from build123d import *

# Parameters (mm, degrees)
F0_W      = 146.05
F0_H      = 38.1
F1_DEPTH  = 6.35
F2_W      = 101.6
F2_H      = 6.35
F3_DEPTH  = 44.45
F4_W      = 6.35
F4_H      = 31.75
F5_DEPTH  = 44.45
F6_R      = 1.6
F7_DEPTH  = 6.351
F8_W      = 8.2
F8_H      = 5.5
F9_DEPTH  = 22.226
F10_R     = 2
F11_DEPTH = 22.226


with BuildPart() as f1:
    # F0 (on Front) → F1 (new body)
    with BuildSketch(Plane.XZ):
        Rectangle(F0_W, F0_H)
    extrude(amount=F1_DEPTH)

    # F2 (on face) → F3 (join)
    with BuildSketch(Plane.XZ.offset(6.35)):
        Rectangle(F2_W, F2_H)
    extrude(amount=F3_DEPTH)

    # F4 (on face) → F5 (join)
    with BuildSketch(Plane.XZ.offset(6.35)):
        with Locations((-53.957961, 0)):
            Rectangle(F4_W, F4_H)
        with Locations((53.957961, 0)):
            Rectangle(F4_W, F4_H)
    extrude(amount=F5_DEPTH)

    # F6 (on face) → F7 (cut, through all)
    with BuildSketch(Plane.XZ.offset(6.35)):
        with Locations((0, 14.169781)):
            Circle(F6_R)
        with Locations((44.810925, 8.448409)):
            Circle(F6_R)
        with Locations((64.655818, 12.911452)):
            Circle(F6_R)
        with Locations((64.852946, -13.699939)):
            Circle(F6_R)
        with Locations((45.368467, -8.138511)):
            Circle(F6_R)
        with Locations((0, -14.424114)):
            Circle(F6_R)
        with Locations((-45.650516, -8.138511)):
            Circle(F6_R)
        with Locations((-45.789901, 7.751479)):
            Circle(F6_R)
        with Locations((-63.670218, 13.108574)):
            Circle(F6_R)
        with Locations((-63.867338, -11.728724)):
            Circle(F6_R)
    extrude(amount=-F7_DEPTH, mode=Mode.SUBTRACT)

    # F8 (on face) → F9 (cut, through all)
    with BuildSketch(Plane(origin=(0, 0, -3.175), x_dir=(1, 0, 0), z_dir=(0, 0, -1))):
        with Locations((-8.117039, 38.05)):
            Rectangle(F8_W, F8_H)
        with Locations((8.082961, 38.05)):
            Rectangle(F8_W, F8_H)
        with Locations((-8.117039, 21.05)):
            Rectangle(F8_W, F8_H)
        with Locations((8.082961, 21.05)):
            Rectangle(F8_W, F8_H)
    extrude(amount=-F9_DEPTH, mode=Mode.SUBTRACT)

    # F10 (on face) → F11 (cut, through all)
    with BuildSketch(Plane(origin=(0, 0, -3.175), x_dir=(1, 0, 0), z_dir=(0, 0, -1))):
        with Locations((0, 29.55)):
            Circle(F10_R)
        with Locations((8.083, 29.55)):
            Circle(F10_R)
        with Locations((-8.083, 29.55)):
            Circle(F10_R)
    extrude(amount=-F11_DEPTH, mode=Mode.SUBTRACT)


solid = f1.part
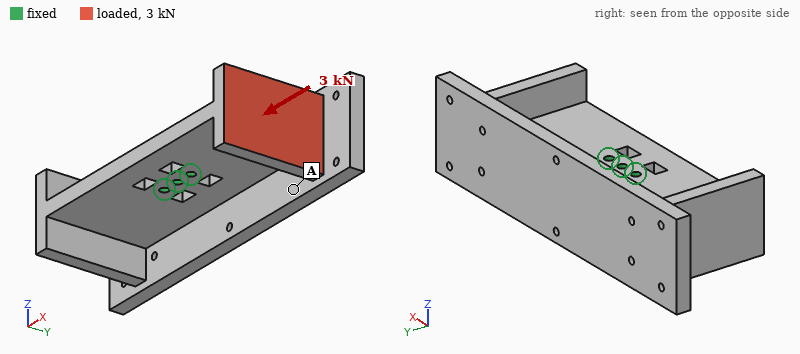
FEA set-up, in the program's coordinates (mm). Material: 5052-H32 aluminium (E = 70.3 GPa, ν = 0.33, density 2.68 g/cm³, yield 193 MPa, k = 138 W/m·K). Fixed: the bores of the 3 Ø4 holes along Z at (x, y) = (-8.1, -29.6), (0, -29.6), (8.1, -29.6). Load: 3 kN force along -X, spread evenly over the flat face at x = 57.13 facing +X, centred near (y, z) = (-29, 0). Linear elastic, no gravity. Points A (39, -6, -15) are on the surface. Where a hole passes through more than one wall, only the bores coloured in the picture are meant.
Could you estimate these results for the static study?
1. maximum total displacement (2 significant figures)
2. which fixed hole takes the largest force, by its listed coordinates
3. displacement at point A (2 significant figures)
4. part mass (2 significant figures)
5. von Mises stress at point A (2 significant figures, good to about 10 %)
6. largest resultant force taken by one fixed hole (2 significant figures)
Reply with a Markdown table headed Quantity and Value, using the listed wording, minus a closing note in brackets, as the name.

| Quantity | Value |
|---|---|
| maximum total displacement | 18 µm |
| which fixed hole takes the largest force, by its listed coordinates | (8.1, -29.6) |
| displacement at point A | 6.5 µm |
| part mass | 210 g |
| von Mises stress at point A | 3.7 MPa |
| largest resultant force taken by one fixed hole | 1.8 kN |
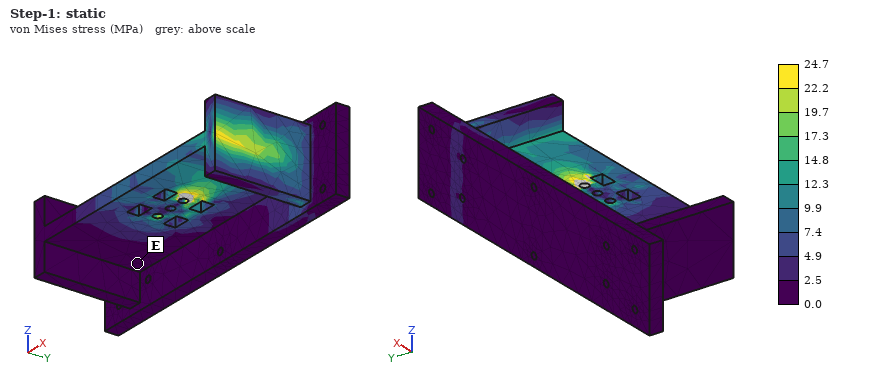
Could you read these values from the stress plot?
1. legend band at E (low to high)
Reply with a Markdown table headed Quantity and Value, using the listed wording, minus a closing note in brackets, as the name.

| Quantity | Value |
|---|---|
| legend band at E | 0.0 to 2.5 MPa |
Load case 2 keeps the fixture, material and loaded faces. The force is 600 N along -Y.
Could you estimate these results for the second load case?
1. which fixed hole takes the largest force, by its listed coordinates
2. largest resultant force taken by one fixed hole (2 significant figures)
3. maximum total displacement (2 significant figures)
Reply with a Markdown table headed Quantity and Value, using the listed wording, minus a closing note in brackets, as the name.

| Quantity | Value |
|---|---|
| which fixed hole takes the largest force, by its listed coordinates | (8.1, -29.6) |
| largest resultant force taken by one fixed hole | 1.8 kN |
| maximum total displacement | 54 µm |
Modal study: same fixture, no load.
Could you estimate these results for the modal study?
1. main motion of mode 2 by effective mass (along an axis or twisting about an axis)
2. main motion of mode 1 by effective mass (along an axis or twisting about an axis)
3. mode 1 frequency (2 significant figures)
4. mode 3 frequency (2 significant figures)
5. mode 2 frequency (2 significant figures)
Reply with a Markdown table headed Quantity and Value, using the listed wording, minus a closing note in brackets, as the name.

| Quantity | Value |
|---|---|
| main motion of mode 2 by effective mass | along Z |
| main motion of mode 1 by effective mass | twisting about Y |
| mode 1 frequency | 900 Hz |
| mode 3 frequency | 1800 Hz |
| mode 2 frequency | 1300 Hz |
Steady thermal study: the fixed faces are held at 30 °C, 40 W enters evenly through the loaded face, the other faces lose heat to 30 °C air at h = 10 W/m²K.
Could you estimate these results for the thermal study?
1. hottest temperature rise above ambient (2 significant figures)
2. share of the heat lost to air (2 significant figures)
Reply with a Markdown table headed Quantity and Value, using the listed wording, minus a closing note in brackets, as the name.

| Quantity | Value |
|---|---|
| hottest temperature rise above ambient | 43 K |
| share of the heat lost to air | 12 % |
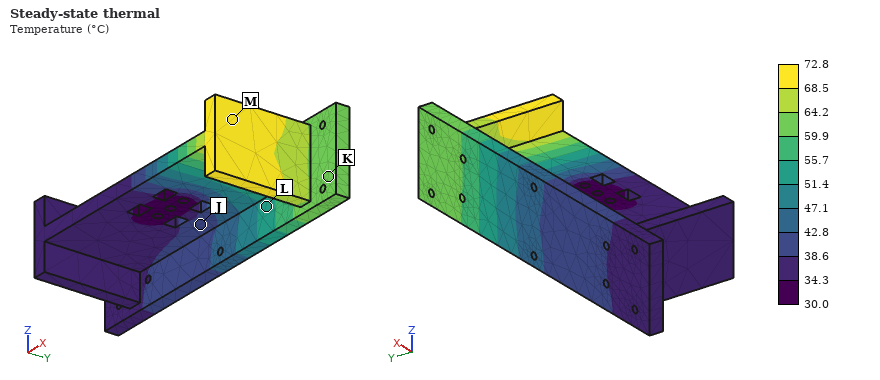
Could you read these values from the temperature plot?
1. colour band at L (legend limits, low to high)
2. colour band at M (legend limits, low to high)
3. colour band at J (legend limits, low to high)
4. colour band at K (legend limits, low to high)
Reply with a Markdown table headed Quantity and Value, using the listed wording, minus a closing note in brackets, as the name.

| Quantity | Value |
|---|---|
| colour band at L | 51.4 to 55.7 °C |
| colour band at M | 68.5 to 72.8 °C |
| colour band at J | 38.6 to 42.8 °C |
| colour band at K | 59.9 to 64.2 °C |
